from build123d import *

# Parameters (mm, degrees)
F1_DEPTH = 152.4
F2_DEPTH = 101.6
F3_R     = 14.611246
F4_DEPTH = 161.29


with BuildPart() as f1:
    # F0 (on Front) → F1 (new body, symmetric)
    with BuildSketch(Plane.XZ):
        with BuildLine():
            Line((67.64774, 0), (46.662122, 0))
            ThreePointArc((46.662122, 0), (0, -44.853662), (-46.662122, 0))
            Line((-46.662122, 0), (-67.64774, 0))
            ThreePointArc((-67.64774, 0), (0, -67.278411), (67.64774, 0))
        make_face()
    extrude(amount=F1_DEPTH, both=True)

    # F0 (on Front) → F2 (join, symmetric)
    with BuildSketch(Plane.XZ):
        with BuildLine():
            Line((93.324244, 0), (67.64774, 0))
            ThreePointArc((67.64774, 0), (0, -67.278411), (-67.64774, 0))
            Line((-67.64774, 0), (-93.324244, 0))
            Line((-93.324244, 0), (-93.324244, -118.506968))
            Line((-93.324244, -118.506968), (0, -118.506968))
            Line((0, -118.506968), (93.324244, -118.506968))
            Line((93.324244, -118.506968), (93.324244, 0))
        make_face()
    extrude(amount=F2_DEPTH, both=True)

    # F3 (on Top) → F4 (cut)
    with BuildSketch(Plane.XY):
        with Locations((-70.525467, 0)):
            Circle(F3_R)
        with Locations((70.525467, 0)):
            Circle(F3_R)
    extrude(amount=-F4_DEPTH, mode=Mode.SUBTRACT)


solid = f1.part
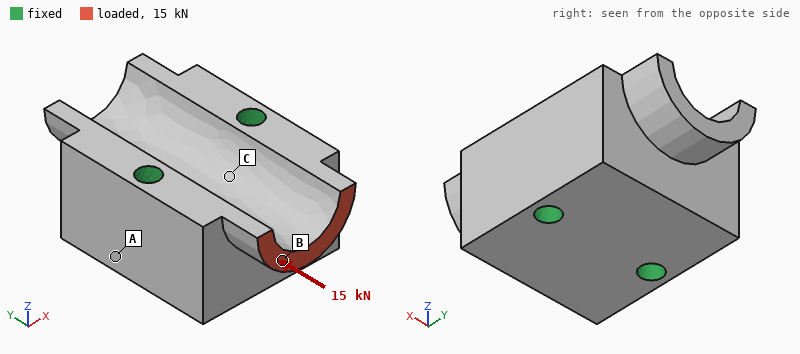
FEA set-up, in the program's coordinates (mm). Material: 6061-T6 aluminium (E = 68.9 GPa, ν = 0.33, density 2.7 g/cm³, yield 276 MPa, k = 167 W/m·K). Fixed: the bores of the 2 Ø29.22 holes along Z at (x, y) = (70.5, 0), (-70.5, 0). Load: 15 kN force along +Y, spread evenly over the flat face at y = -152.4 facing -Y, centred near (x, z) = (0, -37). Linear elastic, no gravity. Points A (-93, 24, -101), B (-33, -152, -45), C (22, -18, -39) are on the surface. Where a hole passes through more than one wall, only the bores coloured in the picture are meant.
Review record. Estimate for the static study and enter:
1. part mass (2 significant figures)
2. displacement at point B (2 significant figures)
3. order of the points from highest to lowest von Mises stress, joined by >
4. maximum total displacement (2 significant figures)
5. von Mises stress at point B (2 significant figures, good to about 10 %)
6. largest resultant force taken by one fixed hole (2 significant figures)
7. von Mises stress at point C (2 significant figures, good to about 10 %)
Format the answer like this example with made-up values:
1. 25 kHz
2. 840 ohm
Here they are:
1. 11 kg
2. 6.2 µm
3. B > C > A
4. 8.7 µm
5. 3.9 MPa
6. 7.7 kN
7. 0.99 MPa
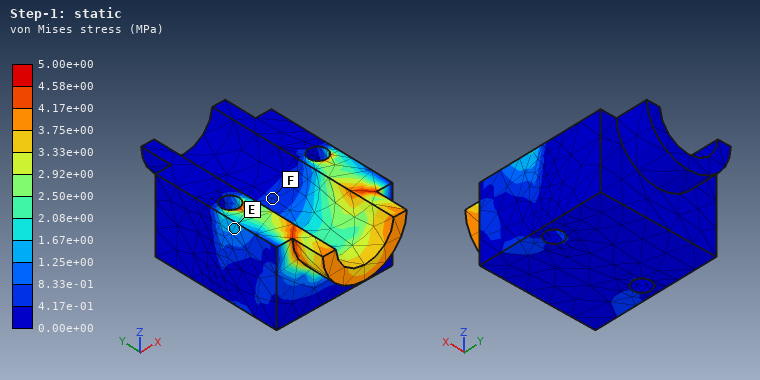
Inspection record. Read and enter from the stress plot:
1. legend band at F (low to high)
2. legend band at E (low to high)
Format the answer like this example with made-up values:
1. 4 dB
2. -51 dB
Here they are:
1. 4.17e-01 to 8.33e-01 MPa
2. 1.25e+00 to 1.67e+00 MPa
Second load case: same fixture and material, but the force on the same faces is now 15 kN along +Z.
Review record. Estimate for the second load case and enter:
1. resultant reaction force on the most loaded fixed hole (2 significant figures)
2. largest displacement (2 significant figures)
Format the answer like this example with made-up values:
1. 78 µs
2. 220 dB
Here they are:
1. 7.5 kN
2. 69 µm
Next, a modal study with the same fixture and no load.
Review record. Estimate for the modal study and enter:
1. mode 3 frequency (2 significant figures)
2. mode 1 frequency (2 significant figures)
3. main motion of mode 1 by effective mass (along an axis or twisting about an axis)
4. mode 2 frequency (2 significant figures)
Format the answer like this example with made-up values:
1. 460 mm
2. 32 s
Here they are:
1. 4400 Hz
2. 4000 Hz
3. twisting about X
4. 4400 Hz
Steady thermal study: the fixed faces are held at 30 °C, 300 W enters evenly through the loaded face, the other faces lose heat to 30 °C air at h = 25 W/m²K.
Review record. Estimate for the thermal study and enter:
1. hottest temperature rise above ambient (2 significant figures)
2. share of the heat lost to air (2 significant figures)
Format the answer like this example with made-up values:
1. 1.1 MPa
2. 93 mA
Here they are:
1. 38 K
2. 8.0 %
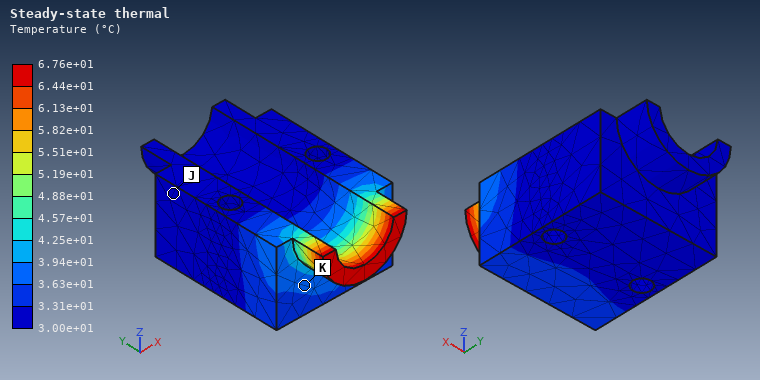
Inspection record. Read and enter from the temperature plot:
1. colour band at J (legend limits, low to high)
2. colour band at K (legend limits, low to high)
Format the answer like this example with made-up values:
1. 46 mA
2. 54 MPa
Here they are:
1. 3.00e+01 to 3.31e+01 °C
2. 3.63e+01 to 3.94e+01 °C
